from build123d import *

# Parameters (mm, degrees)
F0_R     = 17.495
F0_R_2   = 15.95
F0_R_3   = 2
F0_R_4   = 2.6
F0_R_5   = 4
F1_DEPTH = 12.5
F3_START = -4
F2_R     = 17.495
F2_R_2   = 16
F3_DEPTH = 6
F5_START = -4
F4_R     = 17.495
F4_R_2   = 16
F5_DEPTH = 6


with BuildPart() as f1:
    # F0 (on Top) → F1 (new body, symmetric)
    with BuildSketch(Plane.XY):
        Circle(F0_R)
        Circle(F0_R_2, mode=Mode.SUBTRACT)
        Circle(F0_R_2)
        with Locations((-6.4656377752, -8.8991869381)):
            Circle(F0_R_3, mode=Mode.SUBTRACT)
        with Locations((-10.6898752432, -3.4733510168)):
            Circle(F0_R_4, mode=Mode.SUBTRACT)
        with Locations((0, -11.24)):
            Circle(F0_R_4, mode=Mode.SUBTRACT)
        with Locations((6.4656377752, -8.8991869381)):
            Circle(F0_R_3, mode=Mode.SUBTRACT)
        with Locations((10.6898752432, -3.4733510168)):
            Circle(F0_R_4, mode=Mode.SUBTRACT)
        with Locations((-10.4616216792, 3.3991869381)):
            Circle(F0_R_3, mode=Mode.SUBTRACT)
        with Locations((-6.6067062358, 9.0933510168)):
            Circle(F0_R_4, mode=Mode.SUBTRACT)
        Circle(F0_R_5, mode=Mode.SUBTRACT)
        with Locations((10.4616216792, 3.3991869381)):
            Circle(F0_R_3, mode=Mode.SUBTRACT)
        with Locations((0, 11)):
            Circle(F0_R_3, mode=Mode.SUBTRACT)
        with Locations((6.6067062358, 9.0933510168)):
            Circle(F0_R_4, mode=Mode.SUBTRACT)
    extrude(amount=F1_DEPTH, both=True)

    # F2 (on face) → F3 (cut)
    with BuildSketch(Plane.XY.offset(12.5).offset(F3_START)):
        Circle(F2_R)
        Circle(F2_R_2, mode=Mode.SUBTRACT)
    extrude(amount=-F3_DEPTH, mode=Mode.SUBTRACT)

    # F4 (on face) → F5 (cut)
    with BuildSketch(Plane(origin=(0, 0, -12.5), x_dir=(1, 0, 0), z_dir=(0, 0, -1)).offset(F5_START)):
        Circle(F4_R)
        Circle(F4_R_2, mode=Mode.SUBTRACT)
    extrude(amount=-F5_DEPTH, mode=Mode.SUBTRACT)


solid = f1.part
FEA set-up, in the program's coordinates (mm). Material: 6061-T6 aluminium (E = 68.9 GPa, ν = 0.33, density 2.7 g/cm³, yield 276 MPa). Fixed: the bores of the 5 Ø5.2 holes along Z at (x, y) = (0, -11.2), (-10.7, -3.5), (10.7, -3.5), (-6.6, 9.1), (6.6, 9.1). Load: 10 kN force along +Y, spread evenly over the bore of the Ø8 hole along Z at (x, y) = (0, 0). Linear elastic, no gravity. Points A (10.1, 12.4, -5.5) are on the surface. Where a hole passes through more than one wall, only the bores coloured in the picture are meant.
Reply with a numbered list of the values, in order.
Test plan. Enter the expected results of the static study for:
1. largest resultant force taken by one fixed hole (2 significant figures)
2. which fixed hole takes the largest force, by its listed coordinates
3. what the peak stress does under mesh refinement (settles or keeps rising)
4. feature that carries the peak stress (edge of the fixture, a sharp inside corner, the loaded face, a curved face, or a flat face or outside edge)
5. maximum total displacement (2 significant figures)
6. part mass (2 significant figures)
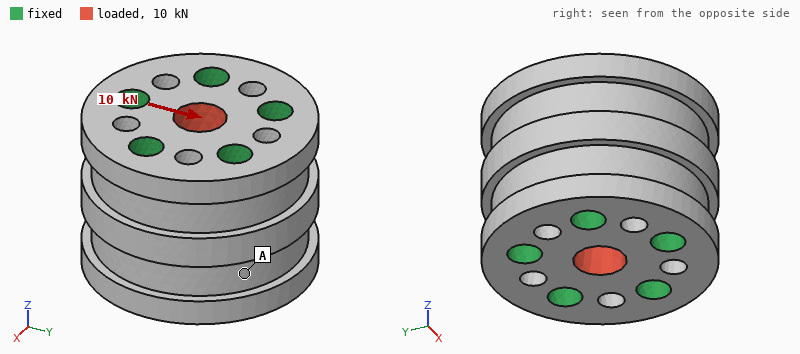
1. 3.3 kN
2. (0, -11.2)
3. keeps rising
4. edge of the fixture
5. 1.7 µm
6. 45 g
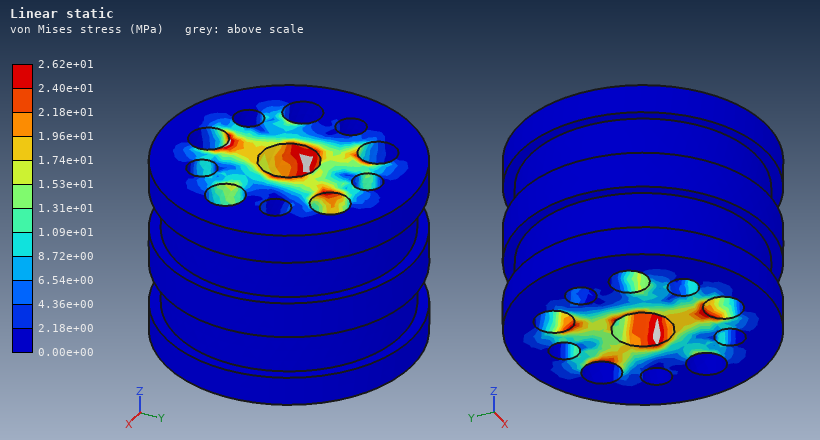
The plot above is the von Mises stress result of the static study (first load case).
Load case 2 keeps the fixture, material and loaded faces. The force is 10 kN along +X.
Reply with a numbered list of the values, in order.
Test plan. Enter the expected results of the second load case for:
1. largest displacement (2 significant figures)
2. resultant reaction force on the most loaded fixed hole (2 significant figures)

1. 1.7 µm
2. 3.1 kN
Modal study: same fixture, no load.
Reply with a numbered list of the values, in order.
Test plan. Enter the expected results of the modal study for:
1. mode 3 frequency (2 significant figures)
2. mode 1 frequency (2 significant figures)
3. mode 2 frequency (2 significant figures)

1. 110 kHz
2. 110 kHz
3. 110 kHz
